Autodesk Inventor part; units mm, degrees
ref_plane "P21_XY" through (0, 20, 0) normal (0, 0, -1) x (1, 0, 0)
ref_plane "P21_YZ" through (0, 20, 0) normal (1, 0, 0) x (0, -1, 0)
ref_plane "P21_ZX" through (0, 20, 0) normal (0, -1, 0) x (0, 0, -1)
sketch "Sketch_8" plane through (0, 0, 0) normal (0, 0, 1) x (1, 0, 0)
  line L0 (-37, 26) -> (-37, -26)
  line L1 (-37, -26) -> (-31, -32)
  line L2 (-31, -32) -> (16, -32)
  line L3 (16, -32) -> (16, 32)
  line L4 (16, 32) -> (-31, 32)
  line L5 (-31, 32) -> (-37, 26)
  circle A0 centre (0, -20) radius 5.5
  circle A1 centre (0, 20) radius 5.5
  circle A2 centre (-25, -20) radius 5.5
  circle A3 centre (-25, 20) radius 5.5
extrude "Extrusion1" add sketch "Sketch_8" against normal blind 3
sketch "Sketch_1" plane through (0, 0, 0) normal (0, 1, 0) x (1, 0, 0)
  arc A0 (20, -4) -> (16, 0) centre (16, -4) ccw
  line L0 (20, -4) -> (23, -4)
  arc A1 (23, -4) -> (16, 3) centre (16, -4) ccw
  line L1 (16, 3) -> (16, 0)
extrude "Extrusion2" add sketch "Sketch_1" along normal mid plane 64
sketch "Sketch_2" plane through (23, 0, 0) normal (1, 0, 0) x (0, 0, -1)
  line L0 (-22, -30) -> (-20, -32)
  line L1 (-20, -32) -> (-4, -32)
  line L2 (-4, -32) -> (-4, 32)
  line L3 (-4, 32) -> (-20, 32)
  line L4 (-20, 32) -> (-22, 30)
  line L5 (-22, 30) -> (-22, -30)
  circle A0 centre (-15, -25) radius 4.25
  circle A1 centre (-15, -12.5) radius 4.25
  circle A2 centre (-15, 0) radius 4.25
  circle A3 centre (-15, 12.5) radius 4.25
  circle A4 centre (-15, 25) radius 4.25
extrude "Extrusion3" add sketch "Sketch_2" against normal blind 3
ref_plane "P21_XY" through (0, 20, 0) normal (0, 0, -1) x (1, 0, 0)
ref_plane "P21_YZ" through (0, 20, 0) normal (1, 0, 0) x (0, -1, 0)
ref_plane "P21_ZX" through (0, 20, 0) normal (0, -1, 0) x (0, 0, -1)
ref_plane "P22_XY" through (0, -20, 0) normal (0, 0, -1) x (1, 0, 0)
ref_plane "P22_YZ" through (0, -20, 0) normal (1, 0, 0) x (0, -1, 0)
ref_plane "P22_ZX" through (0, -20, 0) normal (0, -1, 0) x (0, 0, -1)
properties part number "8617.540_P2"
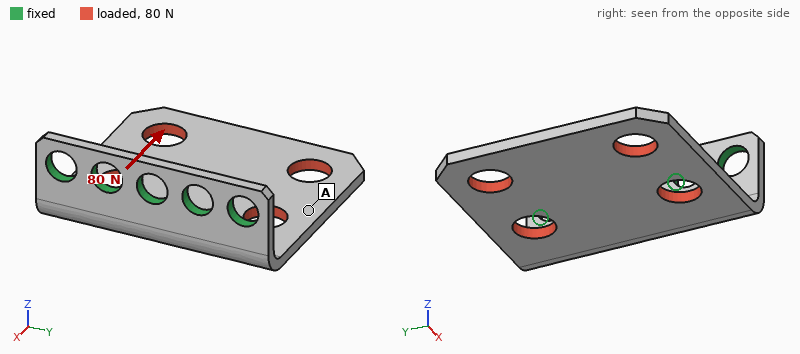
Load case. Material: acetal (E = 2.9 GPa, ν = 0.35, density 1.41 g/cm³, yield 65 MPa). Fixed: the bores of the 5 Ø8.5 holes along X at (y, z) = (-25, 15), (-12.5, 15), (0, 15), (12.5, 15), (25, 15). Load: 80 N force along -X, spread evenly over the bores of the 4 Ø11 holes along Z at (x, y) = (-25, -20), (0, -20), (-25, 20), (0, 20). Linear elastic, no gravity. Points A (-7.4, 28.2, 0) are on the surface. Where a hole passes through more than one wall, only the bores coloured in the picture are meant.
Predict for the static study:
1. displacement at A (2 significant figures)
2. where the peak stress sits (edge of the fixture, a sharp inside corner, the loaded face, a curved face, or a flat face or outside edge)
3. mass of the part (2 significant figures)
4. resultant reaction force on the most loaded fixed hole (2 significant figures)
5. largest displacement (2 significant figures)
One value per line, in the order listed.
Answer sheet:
0.45 mm
a flat face or outside edge
19 g
16 N
0.90 mm
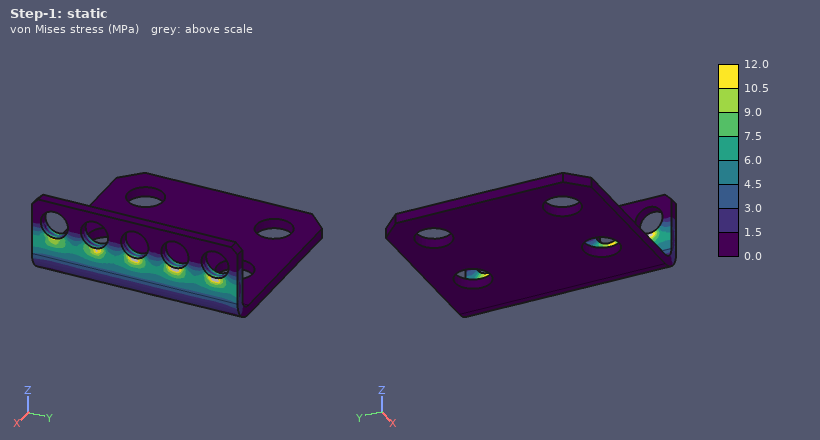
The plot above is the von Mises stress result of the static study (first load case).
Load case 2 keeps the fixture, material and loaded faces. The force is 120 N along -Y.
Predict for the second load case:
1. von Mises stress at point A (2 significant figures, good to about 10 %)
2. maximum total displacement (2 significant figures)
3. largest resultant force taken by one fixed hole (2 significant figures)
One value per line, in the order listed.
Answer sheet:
2.8 MPa
0.99 mm
75 N
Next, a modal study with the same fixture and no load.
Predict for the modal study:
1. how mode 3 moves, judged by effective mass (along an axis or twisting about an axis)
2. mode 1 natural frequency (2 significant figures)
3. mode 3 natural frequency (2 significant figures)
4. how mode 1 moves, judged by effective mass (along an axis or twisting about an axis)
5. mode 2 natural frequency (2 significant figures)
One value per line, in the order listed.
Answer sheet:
along Y
170 Hz
740 Hz
along Z
420 Hz
